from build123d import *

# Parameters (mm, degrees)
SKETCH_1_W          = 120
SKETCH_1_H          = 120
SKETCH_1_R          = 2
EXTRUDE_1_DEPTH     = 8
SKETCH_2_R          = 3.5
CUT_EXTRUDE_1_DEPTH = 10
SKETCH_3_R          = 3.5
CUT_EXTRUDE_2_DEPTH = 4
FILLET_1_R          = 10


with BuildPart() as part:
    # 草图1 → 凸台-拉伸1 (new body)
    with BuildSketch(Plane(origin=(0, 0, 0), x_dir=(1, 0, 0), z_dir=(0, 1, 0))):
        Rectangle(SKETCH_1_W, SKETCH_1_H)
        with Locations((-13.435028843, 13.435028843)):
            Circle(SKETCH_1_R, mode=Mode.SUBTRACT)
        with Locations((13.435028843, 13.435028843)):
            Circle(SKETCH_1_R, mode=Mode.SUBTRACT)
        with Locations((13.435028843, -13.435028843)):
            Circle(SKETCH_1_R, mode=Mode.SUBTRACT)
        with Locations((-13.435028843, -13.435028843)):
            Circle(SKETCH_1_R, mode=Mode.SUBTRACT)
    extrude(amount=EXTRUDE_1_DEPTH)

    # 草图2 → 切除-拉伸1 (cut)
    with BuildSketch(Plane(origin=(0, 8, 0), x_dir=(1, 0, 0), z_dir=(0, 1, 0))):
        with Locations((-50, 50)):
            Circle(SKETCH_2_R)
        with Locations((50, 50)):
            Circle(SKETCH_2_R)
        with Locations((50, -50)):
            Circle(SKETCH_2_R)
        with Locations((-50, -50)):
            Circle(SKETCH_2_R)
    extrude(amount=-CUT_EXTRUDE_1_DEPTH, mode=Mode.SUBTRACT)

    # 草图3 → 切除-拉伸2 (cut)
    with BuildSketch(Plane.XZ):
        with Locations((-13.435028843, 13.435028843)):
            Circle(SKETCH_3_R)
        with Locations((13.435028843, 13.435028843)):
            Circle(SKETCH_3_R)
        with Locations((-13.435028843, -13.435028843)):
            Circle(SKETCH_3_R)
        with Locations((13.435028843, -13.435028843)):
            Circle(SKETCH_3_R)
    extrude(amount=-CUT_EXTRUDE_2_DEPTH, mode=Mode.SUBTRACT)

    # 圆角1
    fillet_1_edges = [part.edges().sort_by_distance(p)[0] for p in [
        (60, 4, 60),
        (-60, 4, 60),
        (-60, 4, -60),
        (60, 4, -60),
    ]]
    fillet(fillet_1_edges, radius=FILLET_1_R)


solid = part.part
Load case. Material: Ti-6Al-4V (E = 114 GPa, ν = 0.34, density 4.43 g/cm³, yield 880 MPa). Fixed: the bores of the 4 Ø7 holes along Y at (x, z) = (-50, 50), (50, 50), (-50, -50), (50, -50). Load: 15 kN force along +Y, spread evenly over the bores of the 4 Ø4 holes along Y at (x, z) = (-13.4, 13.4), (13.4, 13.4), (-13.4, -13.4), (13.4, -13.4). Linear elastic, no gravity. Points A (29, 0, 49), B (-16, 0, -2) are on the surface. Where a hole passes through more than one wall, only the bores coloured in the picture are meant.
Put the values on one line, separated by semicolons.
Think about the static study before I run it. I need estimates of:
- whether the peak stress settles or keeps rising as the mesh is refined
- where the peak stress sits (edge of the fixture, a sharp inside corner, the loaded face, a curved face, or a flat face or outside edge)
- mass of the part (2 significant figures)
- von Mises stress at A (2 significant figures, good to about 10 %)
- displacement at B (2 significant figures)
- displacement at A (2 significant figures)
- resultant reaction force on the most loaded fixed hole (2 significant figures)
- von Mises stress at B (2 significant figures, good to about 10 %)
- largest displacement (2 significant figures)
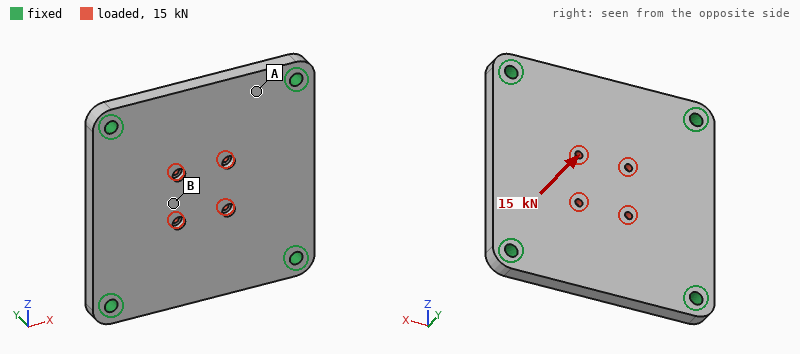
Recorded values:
keeps rising; edge of the fixture; 500 g; 66 MPa; 0.32 mm; 0.066 mm; 3.8 kN; 150 MPa; 0.36 mm
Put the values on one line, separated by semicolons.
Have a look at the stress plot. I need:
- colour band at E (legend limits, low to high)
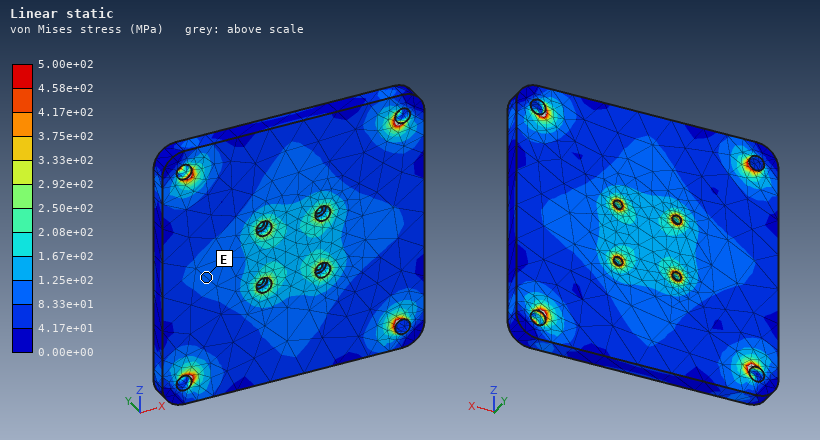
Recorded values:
8.33e+01 to 1.25e+02 MPa
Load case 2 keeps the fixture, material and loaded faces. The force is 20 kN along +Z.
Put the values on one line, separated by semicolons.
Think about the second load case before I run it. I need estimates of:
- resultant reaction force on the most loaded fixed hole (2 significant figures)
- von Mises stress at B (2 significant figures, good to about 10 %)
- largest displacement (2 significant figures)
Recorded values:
5.6 kN; 17 MPa; 21 µm
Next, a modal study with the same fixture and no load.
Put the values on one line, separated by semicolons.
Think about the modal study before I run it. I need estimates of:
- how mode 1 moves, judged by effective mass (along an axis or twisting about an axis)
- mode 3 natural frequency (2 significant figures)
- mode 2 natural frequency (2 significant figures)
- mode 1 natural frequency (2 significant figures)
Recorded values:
along Y; 4500 Hz; 4500 Hz; 2700 Hz
